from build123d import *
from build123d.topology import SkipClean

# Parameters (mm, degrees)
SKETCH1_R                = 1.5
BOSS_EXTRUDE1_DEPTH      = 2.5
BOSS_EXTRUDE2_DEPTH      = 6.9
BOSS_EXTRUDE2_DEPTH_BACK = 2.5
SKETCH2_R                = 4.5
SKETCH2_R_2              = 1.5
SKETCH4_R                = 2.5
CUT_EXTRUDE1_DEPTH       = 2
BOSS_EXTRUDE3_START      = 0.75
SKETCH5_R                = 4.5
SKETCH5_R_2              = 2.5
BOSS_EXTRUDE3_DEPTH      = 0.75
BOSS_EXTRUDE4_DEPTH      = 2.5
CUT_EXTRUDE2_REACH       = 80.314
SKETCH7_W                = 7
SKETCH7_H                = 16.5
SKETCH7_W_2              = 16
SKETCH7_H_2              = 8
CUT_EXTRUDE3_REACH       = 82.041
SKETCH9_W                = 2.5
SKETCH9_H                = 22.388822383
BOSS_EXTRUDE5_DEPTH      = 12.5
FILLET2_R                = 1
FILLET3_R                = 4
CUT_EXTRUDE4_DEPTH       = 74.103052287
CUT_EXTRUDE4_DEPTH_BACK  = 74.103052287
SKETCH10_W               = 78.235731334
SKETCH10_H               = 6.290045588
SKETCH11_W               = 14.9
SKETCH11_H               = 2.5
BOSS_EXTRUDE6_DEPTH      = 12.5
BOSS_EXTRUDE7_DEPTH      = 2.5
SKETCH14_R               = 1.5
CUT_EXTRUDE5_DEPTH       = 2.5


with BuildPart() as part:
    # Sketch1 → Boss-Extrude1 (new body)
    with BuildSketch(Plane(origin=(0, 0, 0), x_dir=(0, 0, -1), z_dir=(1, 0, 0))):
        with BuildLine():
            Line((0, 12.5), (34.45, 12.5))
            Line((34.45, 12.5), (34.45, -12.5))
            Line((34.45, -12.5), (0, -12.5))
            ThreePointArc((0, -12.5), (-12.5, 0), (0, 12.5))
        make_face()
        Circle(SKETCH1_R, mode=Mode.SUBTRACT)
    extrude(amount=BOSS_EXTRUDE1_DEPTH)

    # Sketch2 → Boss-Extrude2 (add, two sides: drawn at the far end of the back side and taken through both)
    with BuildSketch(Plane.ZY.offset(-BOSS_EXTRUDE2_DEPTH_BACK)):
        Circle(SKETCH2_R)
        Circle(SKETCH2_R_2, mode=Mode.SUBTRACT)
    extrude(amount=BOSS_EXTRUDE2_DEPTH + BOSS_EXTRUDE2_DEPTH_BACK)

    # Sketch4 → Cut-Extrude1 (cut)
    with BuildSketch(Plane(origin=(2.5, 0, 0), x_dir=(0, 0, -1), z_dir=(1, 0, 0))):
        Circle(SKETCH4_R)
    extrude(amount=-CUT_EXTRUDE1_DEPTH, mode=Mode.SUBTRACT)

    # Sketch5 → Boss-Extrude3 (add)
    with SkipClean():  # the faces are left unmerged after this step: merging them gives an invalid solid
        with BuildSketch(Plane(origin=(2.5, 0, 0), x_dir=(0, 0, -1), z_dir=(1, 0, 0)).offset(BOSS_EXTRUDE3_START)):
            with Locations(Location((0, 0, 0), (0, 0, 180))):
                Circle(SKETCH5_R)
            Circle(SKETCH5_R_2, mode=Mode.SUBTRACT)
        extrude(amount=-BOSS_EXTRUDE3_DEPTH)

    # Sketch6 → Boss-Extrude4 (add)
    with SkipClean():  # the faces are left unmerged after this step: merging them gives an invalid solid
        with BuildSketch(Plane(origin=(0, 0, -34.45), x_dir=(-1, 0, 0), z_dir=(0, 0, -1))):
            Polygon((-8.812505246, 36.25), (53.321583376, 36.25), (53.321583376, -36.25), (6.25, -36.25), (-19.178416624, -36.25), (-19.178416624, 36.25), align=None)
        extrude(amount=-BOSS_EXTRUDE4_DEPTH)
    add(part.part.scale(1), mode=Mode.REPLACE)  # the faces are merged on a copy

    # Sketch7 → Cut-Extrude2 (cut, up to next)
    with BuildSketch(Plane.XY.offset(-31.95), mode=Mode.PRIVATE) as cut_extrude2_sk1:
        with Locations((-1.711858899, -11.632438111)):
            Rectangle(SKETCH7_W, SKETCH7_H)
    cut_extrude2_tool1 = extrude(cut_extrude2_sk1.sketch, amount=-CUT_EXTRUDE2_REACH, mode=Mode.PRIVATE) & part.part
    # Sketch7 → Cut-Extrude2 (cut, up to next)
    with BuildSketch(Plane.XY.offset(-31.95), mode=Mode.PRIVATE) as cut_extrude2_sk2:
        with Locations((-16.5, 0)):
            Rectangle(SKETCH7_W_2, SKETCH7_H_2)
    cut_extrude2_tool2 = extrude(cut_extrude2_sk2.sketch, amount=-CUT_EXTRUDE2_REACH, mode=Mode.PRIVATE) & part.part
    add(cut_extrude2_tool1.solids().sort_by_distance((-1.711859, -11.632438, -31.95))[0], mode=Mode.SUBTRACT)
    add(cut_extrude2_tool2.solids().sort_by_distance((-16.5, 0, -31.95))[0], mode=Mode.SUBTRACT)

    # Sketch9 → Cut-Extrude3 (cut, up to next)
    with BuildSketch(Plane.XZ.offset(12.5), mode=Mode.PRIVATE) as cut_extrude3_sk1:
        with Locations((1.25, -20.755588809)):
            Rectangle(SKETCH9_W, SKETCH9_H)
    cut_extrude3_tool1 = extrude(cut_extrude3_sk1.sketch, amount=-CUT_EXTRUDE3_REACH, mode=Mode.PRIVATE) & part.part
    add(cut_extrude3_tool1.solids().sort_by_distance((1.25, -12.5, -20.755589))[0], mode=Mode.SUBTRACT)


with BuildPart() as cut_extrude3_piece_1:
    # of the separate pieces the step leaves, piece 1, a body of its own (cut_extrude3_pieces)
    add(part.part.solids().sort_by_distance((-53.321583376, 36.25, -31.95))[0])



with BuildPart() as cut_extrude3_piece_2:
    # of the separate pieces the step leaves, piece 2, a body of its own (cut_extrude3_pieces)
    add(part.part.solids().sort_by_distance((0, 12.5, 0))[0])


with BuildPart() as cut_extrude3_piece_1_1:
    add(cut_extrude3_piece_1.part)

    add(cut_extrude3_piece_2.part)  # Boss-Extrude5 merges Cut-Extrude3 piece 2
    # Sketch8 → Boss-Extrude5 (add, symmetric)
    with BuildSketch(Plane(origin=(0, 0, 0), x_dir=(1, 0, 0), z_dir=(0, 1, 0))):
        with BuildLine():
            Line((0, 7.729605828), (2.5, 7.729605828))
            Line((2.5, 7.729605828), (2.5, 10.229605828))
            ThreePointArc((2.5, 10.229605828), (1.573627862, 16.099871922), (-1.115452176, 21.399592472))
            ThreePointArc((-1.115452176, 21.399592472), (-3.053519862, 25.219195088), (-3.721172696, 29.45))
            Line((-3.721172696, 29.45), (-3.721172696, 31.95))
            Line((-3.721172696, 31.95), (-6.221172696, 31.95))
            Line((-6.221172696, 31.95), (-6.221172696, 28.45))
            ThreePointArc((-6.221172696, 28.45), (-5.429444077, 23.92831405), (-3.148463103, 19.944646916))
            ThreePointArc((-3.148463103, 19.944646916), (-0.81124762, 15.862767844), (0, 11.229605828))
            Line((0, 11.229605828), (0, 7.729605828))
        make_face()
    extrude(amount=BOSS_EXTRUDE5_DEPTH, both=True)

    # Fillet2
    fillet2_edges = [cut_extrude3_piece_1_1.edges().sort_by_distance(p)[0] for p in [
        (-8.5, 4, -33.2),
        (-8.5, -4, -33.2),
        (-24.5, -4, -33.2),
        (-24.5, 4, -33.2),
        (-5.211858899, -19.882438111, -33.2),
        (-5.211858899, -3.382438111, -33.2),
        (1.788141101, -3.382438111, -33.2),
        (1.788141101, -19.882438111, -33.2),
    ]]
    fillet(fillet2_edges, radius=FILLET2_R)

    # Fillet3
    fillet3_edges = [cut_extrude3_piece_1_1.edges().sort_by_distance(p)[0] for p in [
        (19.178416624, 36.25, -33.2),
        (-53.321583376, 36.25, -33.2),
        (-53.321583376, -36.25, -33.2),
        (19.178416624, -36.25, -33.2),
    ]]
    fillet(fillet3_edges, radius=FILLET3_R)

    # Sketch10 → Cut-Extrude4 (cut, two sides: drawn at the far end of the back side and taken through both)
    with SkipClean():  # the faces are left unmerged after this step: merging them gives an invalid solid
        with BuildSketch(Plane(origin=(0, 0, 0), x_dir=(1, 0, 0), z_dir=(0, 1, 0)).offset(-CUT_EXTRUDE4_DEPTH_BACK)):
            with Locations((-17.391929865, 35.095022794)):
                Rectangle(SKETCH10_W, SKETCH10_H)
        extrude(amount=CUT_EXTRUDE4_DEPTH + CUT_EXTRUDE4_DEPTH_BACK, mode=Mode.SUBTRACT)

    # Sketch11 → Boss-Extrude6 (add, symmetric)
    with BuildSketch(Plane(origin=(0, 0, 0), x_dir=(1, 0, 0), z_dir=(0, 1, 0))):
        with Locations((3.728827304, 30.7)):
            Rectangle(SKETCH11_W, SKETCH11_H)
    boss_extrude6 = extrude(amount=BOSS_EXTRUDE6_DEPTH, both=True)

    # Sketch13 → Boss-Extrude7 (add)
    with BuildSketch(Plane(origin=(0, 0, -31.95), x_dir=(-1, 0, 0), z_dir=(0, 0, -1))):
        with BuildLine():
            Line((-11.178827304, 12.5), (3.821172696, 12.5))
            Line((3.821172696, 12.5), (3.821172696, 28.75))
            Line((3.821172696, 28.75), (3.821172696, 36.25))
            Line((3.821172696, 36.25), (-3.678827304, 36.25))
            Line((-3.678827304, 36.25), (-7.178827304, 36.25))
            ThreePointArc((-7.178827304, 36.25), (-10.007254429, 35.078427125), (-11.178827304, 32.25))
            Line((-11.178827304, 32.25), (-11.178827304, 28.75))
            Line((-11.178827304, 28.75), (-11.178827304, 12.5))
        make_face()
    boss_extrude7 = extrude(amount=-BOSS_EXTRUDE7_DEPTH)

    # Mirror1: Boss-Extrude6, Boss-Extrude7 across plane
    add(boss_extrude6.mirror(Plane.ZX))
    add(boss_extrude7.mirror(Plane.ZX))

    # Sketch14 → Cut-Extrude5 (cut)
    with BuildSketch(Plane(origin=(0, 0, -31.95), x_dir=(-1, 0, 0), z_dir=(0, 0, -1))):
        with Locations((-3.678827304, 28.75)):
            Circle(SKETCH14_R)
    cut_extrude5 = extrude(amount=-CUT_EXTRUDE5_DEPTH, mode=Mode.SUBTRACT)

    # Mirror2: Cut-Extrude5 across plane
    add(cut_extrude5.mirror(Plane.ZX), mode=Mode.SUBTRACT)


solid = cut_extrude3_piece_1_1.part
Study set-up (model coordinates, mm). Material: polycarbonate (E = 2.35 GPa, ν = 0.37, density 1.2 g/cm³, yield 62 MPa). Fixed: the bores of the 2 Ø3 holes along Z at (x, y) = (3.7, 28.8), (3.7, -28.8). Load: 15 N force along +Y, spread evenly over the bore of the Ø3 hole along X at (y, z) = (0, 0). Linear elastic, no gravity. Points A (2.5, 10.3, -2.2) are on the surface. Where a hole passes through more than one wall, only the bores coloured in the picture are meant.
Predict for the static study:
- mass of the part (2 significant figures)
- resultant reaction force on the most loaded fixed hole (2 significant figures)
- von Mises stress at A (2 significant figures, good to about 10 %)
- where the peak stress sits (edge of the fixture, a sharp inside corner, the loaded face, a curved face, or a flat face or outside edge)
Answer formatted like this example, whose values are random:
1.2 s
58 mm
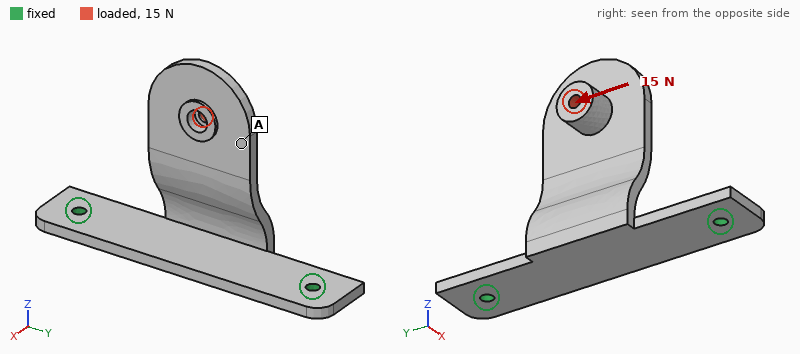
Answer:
6.9 g
14 N
1.7 MPa
a curved face
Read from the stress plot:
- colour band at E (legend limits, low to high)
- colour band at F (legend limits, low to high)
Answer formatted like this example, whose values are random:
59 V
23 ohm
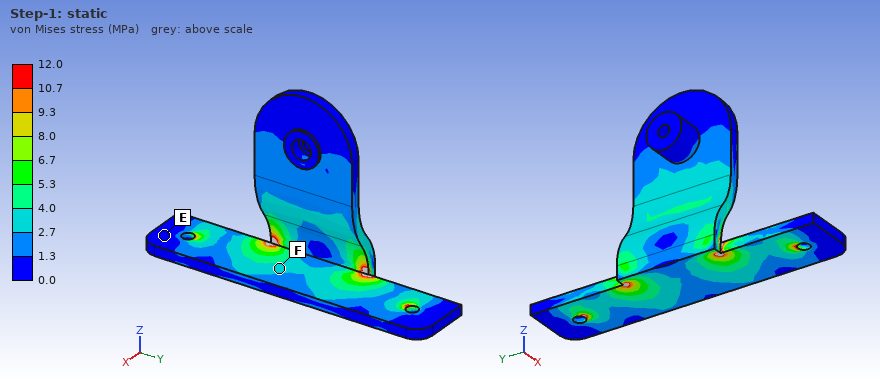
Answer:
0.0 to 1.3 MPa
2.7 to 4.0 MPa
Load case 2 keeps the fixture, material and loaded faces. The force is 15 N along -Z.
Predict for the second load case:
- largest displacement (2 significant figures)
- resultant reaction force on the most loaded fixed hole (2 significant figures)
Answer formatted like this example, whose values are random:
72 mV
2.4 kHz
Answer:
0.92 mm
7.7 N
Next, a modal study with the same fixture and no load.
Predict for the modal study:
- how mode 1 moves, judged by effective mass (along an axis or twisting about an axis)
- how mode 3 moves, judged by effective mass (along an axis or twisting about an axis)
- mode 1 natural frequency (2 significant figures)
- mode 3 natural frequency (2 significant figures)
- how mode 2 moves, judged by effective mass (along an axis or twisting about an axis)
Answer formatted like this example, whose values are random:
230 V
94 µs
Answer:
along X
along Z
190 Hz
660 Hz
along Y
